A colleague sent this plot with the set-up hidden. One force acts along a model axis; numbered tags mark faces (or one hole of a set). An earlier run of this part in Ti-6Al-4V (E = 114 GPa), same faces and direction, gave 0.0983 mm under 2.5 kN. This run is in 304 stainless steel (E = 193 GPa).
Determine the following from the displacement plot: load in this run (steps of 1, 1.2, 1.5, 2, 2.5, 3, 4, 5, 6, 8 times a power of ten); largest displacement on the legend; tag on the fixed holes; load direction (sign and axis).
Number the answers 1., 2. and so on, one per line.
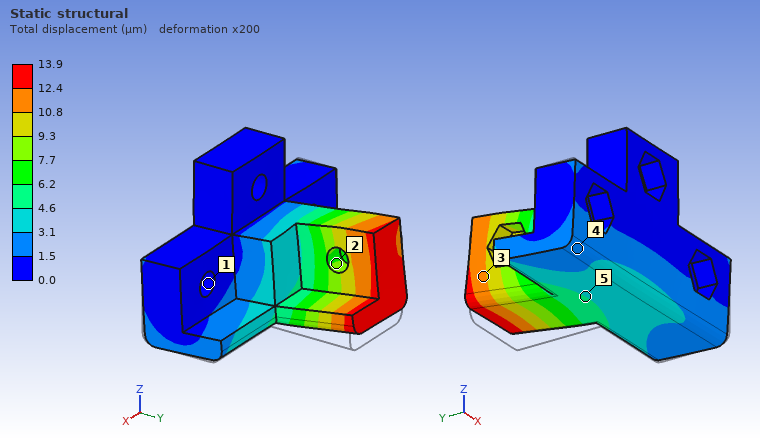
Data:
1. 600 N
2. 13.9 µm
3. 1
4. +Z
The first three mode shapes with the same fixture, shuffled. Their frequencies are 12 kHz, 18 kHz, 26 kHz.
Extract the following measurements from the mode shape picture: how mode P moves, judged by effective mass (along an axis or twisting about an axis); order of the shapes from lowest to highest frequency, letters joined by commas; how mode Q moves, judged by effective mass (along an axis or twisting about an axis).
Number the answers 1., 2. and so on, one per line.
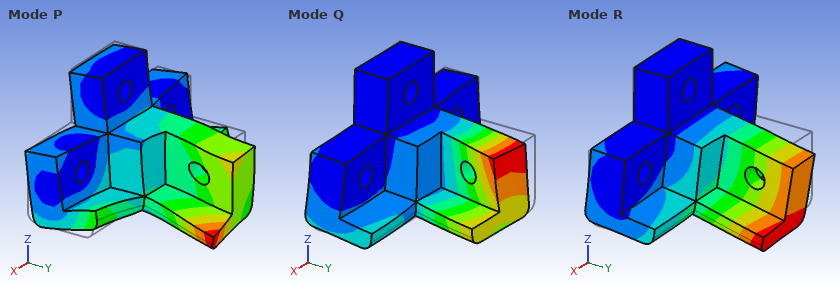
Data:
1. along Y
2. R, Q, P
3. along X
